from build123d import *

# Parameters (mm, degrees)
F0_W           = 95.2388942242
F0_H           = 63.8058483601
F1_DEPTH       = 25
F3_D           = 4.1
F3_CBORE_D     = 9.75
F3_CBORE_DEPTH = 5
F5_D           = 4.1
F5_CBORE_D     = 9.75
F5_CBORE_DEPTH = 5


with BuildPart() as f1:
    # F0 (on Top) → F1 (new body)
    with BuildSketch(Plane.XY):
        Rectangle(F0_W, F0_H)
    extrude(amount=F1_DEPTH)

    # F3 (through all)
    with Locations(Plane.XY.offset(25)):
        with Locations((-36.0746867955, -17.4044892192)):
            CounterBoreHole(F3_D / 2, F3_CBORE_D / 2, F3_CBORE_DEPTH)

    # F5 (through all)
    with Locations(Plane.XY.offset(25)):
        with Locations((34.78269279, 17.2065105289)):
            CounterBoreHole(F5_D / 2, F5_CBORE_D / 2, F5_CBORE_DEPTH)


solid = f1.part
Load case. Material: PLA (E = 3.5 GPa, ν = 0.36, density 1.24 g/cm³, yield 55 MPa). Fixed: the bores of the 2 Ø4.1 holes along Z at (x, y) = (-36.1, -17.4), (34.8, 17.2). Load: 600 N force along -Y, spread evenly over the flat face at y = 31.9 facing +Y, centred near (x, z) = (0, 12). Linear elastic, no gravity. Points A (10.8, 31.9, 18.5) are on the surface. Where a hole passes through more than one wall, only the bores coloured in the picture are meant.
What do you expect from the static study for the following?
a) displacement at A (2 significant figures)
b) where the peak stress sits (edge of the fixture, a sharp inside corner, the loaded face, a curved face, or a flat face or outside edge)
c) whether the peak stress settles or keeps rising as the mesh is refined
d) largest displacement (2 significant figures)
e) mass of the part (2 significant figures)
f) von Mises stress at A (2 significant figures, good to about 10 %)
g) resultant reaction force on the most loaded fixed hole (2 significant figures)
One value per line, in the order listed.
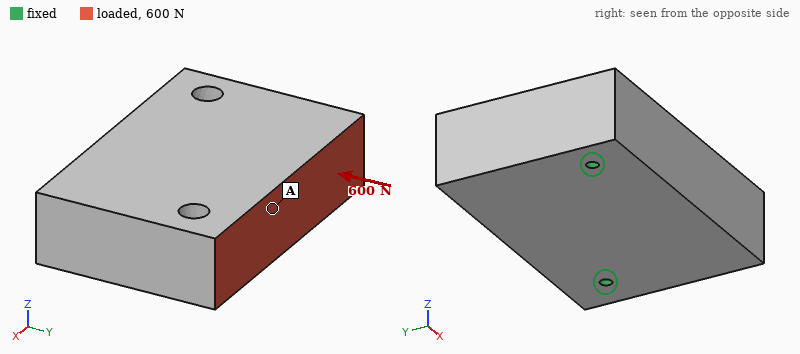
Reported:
7.0 µm
edge of the fixture
keeps rising
8.9 µm
190 g
0.26 MPa
300 N
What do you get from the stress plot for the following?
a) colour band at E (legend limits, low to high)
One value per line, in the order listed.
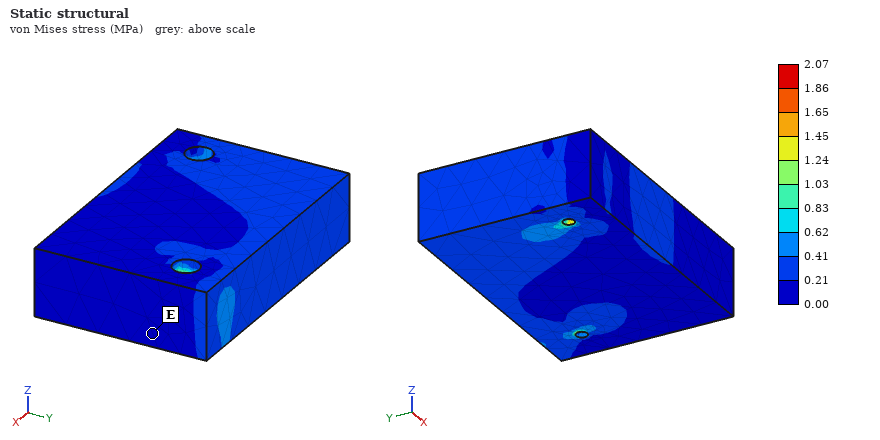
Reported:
0.00 to 0.21 MPa
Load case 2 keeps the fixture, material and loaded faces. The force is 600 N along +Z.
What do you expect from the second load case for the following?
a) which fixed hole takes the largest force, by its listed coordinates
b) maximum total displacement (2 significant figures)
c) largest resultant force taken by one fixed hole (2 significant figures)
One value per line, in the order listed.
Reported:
(34.8, 17.2)
0.12 mm
410 N
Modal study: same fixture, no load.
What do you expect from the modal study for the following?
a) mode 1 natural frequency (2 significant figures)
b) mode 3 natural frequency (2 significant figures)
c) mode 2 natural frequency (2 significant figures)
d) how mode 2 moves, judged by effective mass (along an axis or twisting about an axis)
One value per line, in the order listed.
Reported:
1600 Hz
3800 Hz
2300 Hz
along Z
